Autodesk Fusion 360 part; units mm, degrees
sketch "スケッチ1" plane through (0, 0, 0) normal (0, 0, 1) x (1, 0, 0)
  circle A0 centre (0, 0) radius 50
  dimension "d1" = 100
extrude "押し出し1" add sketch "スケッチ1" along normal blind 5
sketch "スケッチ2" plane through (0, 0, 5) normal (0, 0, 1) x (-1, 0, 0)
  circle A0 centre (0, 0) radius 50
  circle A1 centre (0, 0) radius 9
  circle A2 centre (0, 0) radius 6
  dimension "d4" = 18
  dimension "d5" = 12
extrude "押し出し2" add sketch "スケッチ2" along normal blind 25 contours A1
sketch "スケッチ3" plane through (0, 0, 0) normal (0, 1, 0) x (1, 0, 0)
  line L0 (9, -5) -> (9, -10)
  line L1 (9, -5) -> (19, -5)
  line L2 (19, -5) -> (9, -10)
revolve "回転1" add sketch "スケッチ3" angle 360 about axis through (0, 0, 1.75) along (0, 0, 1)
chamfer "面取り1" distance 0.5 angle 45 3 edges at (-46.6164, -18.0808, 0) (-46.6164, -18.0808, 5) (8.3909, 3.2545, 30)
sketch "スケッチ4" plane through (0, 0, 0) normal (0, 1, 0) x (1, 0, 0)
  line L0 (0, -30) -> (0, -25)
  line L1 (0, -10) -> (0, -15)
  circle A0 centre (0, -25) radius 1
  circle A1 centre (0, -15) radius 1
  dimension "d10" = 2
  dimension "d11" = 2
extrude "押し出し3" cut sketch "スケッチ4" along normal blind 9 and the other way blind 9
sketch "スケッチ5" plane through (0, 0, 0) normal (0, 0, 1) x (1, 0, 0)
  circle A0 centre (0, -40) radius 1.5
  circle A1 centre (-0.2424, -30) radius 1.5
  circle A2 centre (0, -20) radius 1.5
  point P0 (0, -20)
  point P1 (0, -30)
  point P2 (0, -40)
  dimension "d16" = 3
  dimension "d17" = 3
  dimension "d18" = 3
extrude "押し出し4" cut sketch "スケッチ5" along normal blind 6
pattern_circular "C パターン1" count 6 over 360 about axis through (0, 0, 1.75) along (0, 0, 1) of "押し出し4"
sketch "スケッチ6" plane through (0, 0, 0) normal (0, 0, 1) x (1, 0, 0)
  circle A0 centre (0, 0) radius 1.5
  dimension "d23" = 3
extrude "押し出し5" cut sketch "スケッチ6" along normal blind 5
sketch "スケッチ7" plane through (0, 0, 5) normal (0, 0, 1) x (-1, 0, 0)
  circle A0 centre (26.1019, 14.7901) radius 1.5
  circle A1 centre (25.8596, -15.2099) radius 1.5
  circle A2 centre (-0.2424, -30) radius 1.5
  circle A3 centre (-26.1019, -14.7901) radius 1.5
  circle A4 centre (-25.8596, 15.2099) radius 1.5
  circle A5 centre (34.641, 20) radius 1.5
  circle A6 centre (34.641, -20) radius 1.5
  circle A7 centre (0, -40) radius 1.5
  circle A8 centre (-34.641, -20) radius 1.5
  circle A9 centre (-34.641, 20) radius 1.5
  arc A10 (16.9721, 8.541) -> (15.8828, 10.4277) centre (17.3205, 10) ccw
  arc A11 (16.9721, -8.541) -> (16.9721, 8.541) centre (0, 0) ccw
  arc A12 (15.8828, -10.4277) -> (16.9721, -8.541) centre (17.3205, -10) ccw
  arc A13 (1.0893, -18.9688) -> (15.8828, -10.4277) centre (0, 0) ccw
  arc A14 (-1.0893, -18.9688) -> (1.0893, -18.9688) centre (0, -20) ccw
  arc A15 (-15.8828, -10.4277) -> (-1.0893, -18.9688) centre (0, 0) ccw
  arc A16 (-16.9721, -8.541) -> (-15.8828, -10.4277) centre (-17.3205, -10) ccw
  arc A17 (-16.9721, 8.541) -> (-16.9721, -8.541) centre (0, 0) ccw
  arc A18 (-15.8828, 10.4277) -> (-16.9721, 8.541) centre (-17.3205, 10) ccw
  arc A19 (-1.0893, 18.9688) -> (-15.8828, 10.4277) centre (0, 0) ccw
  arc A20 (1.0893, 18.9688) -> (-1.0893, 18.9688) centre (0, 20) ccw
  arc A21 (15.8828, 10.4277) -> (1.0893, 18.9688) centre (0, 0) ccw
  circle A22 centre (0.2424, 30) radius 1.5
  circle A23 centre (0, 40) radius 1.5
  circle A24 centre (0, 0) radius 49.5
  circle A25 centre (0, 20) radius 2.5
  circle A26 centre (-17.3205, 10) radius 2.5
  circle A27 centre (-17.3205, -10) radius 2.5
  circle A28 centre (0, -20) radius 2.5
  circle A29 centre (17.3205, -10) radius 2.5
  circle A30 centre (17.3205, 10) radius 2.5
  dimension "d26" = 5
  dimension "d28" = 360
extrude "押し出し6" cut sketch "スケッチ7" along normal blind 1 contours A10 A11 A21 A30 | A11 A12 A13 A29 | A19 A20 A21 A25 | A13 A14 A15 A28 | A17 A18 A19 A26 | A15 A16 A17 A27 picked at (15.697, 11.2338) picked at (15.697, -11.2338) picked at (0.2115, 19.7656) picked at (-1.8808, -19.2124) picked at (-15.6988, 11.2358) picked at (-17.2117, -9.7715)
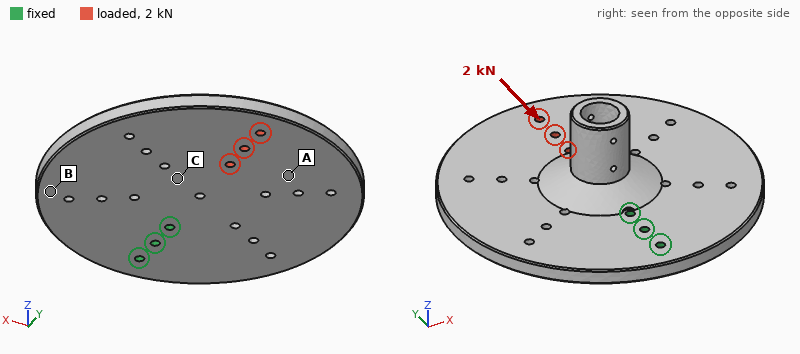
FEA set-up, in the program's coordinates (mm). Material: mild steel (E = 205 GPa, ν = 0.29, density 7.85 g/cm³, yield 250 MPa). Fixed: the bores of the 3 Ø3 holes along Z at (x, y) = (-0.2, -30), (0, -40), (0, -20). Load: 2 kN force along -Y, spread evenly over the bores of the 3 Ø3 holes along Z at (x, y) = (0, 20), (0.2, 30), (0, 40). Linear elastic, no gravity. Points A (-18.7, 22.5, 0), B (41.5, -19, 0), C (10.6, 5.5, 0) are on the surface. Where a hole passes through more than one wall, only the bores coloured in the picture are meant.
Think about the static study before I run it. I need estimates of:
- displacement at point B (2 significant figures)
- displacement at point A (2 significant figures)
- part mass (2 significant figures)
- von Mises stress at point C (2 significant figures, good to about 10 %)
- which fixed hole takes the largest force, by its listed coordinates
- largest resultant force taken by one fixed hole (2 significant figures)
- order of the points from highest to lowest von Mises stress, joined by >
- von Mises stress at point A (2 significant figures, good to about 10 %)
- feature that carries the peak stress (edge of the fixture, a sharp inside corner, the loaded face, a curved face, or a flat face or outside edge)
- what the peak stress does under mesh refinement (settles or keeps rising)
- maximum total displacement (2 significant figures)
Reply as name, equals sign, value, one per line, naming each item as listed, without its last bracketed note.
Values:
displacement at point B = 2.1 µm
displacement at point A = 3.7 µm
part mass = 340 g
von Mises stress at point C = 11 MPa
which fixed hole takes the largest force, by its listed coordinates = (0, -20)
largest resultant force taken by one fixed hole = 1.2 kN
order of the points from highest to lowest von Mises stress, joined by > = C > A > B
von Mises stress at point A = 4.6 MPa
feature that carries the peak stress = edge of the fixture
what the peak stress does under mesh refinement = keeps rising
maximum total displacement = 8.1 µm
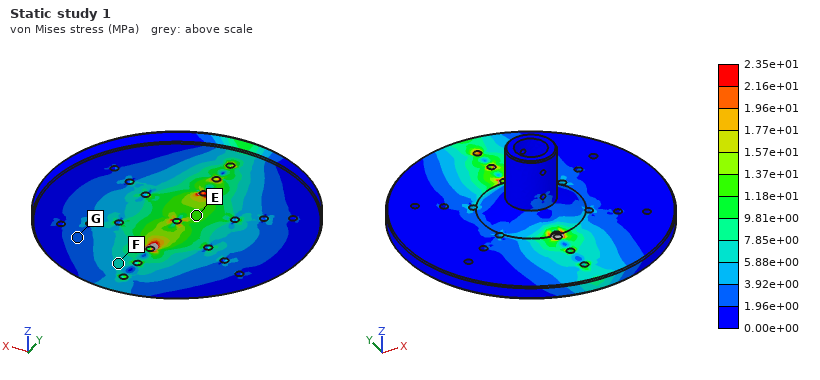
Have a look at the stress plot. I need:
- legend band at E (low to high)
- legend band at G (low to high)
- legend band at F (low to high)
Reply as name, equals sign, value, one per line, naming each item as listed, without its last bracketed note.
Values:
legend band at E = 1.18e+01 to 1.37e+01 MPa
legend band at G = 1.96e+00 to 3.92e+00 MPa
legend band at F = 5.88e+00 to 7.85e+00 MPa
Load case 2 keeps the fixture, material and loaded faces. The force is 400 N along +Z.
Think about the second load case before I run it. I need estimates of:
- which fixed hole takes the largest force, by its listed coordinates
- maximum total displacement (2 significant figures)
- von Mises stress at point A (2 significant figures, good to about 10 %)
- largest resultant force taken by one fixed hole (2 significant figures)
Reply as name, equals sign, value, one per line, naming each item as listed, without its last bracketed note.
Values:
which fixed hole takes the largest force, by its listed coordinates = (0, -20)
maximum total displacement = 0.15 mm
von Mises stress at point A = 12 MPa
largest resultant force taken by one fixed hole = 1.2 kN
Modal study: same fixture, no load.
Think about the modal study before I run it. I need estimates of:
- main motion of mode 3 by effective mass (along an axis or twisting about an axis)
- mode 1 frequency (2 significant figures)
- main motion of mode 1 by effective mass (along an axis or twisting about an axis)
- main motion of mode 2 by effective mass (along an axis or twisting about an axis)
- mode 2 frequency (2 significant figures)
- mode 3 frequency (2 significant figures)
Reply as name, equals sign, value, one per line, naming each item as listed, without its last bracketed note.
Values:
main motion of mode 3 by effective mass = along Z
mode 1 frequency = 930 Hz
main motion of mode 1 by effective mass = along Z
main motion of mode 2 by effective mass = twisting about Y
mode 2 frequency = 1200 Hz
mode 3 frequency = 2900 Hz
